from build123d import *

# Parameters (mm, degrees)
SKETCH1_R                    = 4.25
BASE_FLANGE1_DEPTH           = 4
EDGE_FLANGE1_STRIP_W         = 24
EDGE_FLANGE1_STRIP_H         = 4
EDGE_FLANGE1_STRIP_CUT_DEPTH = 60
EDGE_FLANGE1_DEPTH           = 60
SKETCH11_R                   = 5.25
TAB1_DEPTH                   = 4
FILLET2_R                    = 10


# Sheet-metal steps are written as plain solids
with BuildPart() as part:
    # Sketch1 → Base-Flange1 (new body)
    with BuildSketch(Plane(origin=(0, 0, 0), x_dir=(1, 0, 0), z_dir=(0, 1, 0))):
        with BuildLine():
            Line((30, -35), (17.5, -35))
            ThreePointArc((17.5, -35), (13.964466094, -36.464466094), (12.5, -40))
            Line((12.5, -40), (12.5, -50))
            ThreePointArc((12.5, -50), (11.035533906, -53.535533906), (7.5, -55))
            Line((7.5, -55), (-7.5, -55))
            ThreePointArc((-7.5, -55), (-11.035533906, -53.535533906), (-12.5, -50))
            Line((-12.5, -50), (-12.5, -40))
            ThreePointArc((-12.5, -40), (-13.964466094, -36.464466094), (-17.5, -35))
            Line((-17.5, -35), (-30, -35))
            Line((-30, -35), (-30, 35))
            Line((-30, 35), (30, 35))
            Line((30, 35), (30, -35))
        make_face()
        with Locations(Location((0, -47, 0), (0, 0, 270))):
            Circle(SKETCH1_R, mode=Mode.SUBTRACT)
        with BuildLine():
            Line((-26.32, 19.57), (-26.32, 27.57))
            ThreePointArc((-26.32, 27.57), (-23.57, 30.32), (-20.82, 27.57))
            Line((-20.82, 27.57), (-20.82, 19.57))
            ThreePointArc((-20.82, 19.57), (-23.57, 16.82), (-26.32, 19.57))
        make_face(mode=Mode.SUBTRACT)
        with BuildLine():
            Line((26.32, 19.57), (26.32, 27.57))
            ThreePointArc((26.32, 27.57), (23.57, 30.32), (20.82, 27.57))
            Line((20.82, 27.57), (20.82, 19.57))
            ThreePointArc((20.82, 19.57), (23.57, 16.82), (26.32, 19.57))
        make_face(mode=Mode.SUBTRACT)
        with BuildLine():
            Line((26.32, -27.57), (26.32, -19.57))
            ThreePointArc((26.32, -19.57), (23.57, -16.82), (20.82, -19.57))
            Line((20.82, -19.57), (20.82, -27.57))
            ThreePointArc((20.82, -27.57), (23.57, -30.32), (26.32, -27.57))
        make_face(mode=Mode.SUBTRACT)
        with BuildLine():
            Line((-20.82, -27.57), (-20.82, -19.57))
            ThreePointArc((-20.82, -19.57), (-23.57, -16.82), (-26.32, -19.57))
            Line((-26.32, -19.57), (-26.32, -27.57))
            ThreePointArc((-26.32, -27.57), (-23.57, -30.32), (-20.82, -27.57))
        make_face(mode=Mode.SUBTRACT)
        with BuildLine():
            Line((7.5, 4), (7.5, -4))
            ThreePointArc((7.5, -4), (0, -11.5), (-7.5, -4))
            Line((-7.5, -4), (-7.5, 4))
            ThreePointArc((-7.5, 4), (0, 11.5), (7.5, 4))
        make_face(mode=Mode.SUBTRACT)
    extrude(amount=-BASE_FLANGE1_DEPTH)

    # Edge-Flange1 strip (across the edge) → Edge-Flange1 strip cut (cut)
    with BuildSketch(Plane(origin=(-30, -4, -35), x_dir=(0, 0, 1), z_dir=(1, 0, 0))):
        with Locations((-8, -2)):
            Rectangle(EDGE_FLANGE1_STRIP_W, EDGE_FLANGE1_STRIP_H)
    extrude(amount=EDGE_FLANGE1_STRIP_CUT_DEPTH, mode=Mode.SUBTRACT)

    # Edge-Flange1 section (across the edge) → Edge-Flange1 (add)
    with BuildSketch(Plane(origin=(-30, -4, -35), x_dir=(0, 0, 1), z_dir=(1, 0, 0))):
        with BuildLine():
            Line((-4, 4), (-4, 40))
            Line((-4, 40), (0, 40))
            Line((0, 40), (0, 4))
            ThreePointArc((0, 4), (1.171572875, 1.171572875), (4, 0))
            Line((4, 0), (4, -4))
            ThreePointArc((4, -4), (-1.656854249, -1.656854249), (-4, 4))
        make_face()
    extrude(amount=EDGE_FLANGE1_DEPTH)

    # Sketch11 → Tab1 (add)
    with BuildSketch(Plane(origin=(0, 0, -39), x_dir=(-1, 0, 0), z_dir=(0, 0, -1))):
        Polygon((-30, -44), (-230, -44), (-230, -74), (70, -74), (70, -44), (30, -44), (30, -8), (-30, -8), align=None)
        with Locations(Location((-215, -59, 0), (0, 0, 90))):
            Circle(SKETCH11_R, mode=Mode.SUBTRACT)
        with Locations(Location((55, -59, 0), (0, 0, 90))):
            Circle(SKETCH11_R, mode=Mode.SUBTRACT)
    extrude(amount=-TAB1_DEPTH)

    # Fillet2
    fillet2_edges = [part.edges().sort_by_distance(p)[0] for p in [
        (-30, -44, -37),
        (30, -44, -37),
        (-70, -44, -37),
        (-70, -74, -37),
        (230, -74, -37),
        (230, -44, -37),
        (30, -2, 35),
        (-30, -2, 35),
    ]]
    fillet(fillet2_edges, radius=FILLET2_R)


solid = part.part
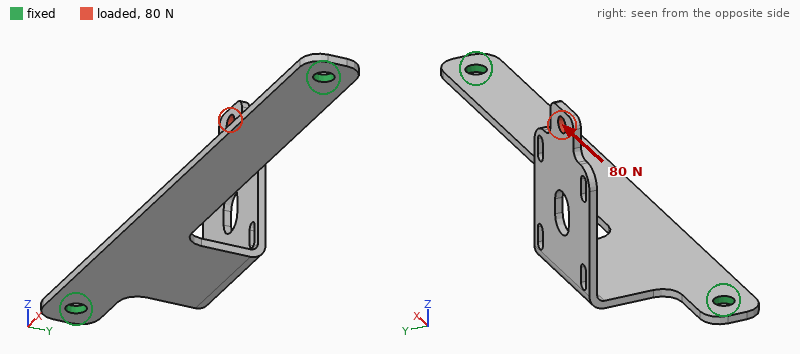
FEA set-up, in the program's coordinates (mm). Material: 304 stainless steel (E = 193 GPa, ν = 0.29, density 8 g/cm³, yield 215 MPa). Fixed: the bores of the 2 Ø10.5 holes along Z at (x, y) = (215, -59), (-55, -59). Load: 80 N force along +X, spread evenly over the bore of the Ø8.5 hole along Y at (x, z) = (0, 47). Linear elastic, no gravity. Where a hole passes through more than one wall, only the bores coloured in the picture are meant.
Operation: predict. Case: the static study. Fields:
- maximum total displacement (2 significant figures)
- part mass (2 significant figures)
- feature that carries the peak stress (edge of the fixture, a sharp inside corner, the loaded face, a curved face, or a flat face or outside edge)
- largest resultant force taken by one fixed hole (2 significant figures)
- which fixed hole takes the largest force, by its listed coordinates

0.54 mm
490 g
a flat face or outside edge
70 N
(-55, -59)
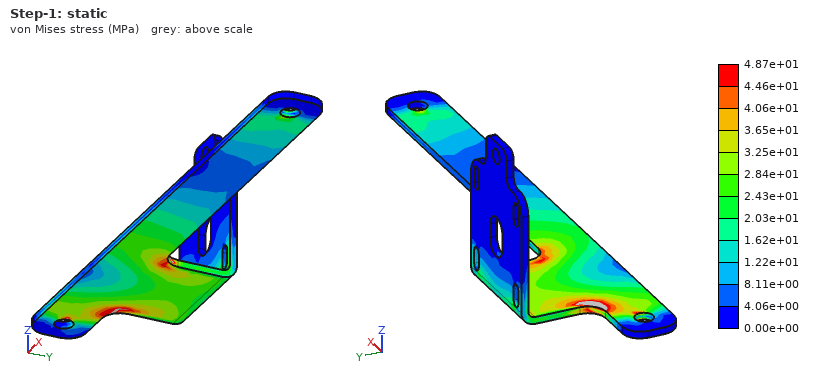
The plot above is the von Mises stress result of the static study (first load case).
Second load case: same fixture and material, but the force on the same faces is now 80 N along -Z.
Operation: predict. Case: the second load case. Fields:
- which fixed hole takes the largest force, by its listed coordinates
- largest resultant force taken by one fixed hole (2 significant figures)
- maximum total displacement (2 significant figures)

(-55, -59)
71 N
0.49 mm
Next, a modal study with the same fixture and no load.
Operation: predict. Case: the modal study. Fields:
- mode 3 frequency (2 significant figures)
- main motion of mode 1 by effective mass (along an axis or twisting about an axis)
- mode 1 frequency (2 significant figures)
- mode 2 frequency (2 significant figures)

480 Hz
along Z
170 Hz
230 Hz
